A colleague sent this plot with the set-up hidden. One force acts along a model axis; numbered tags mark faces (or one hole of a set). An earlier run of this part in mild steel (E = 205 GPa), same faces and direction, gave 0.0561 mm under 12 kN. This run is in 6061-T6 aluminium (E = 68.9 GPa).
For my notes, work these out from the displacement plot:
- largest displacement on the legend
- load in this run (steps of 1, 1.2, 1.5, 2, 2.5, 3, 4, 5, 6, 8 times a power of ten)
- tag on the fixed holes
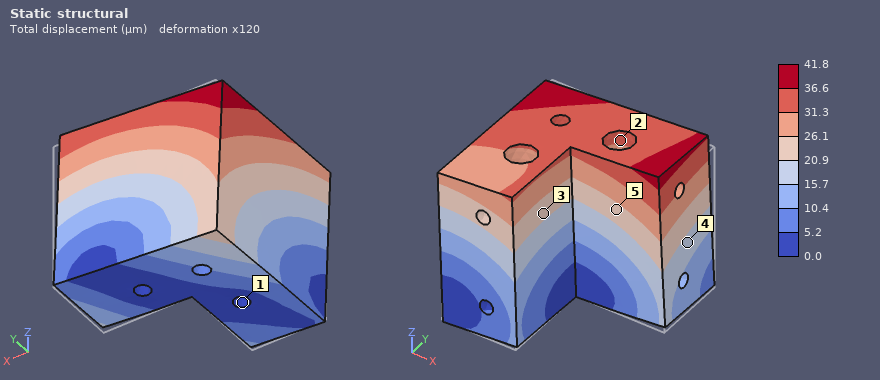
41.8 µm
3 kN
1
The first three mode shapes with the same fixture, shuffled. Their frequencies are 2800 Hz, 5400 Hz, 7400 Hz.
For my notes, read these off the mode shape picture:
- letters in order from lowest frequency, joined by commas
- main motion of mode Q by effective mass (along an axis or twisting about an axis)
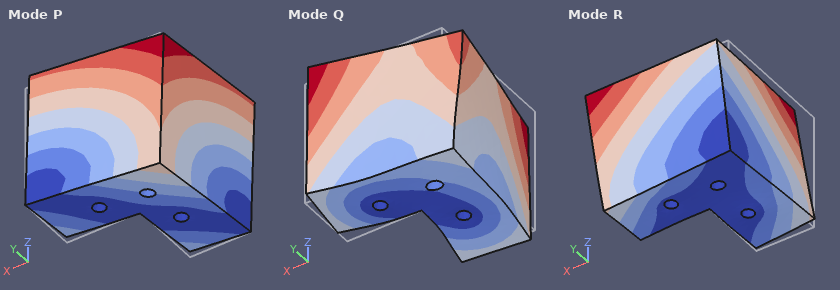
P, R, Q
twisting about Z
